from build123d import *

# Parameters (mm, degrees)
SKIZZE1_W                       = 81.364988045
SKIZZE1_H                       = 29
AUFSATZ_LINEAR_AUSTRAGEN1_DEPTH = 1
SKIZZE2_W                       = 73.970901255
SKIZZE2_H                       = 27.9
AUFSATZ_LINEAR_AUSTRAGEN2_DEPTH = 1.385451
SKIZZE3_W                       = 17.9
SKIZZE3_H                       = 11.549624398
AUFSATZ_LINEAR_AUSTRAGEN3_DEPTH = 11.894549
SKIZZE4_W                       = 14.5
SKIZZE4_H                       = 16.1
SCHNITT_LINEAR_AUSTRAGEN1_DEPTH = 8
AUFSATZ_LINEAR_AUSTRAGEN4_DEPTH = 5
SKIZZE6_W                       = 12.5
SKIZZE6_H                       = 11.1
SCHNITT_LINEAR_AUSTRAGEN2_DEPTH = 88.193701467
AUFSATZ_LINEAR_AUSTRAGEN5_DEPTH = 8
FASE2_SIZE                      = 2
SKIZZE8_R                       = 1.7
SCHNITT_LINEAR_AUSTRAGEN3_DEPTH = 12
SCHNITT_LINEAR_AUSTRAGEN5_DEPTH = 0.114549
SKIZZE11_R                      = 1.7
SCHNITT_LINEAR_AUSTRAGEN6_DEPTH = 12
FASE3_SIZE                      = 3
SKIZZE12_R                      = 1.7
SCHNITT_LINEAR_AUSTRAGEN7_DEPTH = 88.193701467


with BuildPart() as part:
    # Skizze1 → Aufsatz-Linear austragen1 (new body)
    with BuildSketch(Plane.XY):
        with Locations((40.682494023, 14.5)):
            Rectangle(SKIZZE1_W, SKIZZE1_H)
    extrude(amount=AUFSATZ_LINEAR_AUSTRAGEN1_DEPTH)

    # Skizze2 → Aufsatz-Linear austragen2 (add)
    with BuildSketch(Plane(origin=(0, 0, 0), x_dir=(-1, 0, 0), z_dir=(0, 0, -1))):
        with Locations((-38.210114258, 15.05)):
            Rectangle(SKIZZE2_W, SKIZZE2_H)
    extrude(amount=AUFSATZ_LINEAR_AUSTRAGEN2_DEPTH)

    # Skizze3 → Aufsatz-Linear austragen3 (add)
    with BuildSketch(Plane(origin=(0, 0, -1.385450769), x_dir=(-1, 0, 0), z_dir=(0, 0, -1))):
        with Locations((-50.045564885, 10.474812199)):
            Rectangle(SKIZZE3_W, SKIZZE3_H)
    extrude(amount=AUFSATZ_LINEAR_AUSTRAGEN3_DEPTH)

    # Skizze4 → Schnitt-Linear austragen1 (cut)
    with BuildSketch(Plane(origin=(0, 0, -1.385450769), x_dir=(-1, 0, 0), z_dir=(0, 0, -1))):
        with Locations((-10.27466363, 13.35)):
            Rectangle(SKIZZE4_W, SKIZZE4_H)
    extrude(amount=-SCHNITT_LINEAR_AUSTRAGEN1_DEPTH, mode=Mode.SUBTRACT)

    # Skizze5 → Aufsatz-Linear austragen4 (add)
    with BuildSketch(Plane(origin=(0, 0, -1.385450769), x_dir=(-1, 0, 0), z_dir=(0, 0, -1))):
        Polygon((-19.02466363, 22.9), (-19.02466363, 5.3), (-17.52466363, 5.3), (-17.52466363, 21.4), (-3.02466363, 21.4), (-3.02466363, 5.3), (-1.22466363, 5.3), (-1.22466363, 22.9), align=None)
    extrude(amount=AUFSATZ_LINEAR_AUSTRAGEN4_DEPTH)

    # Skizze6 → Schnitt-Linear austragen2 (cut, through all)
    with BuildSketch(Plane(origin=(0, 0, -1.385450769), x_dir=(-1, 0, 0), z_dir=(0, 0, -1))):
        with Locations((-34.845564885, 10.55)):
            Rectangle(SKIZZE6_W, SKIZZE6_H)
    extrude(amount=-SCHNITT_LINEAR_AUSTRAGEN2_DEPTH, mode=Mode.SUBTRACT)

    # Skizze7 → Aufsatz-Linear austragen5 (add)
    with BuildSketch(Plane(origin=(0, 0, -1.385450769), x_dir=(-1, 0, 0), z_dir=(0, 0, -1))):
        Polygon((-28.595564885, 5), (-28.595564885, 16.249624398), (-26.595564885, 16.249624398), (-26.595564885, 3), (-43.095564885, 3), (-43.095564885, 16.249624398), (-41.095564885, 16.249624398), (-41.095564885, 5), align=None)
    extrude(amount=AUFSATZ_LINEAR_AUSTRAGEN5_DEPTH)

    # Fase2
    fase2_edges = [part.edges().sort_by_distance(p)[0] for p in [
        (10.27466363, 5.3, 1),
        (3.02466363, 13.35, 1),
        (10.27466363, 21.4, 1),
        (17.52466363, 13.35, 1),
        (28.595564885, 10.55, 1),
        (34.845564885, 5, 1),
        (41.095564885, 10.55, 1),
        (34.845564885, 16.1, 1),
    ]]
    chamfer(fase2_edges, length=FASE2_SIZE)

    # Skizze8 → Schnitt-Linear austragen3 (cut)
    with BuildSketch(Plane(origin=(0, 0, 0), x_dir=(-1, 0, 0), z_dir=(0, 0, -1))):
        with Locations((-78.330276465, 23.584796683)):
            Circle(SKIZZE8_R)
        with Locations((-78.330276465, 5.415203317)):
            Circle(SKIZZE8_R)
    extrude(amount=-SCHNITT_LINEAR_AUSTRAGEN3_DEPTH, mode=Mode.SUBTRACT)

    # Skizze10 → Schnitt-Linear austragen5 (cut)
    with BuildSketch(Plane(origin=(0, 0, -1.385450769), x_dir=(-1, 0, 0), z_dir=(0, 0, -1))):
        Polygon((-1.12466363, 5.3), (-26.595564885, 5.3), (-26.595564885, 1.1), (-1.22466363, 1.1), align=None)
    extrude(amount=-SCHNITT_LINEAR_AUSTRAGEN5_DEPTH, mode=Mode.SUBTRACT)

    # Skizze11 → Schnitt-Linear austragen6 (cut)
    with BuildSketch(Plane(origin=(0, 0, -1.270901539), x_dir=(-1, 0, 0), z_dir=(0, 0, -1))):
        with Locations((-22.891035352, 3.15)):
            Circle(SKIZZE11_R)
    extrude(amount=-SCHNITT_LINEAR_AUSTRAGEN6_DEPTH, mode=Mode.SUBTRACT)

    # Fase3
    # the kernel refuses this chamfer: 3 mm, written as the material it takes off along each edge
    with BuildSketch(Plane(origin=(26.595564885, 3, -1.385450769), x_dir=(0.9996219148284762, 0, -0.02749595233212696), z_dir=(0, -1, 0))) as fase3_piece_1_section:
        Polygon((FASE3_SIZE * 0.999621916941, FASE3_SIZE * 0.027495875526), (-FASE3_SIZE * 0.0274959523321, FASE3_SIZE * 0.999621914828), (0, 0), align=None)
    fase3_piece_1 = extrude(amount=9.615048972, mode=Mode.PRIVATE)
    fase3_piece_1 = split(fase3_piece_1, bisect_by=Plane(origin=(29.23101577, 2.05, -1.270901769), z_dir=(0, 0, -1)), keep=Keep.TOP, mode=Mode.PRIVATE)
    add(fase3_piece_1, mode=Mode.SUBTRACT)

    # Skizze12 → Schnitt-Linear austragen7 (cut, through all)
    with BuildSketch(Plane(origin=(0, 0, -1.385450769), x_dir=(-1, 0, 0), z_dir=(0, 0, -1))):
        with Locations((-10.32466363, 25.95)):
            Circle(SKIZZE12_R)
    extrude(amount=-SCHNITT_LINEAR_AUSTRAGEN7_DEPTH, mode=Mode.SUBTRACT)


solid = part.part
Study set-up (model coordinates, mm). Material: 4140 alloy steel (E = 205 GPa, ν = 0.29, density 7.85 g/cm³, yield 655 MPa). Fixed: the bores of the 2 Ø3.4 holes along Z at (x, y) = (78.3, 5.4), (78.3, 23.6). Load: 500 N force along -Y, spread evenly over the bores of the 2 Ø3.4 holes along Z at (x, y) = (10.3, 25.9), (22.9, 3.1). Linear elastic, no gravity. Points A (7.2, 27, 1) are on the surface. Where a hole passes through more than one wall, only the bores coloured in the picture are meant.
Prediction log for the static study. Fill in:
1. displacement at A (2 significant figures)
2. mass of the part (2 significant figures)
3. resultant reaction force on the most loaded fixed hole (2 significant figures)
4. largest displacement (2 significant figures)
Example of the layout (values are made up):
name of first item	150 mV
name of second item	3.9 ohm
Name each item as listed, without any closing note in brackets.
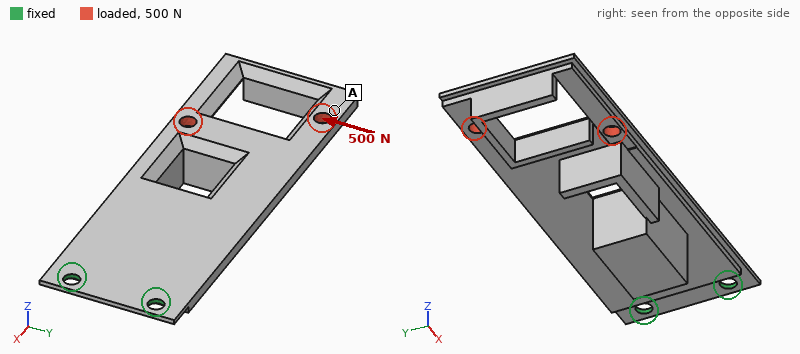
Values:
displacement at A	0.13 mm
mass of the part	57 g
resultant reaction force on the most loaded fixed hole	1.6 kN
largest displacement	0.16 mm
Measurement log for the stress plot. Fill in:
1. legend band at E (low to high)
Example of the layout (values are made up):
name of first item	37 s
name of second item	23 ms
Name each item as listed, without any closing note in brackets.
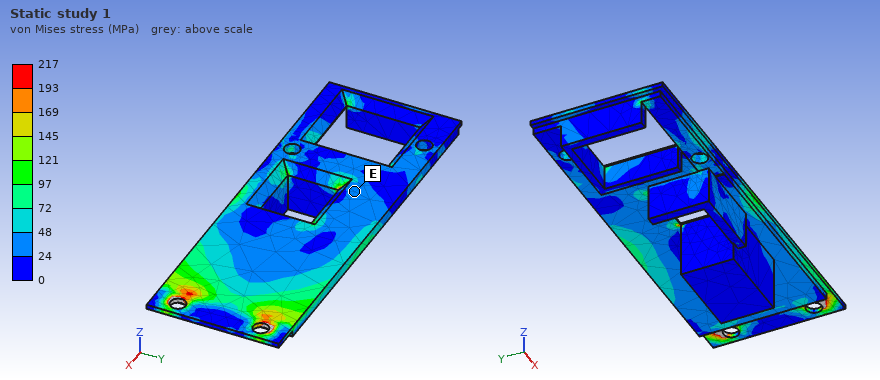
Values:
legend band at E	24 to 48 MPa
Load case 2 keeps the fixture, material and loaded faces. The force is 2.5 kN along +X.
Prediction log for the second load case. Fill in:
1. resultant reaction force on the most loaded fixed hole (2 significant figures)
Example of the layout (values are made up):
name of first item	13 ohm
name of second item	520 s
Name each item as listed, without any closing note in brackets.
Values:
resultant reaction force on the most loaded fixed hole	1.3 kN
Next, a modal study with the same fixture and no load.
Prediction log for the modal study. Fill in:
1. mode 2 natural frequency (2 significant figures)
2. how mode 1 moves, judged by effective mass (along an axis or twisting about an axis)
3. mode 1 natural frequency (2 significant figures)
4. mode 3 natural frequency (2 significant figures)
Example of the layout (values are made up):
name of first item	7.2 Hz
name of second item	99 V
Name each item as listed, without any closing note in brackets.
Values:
mode 2 natural frequency	1600 Hz
how mode 1 moves, judged by effective mass	along Z
mode 1 natural frequency	210 Hz
mode 3 natural frequency	2000 Hz
